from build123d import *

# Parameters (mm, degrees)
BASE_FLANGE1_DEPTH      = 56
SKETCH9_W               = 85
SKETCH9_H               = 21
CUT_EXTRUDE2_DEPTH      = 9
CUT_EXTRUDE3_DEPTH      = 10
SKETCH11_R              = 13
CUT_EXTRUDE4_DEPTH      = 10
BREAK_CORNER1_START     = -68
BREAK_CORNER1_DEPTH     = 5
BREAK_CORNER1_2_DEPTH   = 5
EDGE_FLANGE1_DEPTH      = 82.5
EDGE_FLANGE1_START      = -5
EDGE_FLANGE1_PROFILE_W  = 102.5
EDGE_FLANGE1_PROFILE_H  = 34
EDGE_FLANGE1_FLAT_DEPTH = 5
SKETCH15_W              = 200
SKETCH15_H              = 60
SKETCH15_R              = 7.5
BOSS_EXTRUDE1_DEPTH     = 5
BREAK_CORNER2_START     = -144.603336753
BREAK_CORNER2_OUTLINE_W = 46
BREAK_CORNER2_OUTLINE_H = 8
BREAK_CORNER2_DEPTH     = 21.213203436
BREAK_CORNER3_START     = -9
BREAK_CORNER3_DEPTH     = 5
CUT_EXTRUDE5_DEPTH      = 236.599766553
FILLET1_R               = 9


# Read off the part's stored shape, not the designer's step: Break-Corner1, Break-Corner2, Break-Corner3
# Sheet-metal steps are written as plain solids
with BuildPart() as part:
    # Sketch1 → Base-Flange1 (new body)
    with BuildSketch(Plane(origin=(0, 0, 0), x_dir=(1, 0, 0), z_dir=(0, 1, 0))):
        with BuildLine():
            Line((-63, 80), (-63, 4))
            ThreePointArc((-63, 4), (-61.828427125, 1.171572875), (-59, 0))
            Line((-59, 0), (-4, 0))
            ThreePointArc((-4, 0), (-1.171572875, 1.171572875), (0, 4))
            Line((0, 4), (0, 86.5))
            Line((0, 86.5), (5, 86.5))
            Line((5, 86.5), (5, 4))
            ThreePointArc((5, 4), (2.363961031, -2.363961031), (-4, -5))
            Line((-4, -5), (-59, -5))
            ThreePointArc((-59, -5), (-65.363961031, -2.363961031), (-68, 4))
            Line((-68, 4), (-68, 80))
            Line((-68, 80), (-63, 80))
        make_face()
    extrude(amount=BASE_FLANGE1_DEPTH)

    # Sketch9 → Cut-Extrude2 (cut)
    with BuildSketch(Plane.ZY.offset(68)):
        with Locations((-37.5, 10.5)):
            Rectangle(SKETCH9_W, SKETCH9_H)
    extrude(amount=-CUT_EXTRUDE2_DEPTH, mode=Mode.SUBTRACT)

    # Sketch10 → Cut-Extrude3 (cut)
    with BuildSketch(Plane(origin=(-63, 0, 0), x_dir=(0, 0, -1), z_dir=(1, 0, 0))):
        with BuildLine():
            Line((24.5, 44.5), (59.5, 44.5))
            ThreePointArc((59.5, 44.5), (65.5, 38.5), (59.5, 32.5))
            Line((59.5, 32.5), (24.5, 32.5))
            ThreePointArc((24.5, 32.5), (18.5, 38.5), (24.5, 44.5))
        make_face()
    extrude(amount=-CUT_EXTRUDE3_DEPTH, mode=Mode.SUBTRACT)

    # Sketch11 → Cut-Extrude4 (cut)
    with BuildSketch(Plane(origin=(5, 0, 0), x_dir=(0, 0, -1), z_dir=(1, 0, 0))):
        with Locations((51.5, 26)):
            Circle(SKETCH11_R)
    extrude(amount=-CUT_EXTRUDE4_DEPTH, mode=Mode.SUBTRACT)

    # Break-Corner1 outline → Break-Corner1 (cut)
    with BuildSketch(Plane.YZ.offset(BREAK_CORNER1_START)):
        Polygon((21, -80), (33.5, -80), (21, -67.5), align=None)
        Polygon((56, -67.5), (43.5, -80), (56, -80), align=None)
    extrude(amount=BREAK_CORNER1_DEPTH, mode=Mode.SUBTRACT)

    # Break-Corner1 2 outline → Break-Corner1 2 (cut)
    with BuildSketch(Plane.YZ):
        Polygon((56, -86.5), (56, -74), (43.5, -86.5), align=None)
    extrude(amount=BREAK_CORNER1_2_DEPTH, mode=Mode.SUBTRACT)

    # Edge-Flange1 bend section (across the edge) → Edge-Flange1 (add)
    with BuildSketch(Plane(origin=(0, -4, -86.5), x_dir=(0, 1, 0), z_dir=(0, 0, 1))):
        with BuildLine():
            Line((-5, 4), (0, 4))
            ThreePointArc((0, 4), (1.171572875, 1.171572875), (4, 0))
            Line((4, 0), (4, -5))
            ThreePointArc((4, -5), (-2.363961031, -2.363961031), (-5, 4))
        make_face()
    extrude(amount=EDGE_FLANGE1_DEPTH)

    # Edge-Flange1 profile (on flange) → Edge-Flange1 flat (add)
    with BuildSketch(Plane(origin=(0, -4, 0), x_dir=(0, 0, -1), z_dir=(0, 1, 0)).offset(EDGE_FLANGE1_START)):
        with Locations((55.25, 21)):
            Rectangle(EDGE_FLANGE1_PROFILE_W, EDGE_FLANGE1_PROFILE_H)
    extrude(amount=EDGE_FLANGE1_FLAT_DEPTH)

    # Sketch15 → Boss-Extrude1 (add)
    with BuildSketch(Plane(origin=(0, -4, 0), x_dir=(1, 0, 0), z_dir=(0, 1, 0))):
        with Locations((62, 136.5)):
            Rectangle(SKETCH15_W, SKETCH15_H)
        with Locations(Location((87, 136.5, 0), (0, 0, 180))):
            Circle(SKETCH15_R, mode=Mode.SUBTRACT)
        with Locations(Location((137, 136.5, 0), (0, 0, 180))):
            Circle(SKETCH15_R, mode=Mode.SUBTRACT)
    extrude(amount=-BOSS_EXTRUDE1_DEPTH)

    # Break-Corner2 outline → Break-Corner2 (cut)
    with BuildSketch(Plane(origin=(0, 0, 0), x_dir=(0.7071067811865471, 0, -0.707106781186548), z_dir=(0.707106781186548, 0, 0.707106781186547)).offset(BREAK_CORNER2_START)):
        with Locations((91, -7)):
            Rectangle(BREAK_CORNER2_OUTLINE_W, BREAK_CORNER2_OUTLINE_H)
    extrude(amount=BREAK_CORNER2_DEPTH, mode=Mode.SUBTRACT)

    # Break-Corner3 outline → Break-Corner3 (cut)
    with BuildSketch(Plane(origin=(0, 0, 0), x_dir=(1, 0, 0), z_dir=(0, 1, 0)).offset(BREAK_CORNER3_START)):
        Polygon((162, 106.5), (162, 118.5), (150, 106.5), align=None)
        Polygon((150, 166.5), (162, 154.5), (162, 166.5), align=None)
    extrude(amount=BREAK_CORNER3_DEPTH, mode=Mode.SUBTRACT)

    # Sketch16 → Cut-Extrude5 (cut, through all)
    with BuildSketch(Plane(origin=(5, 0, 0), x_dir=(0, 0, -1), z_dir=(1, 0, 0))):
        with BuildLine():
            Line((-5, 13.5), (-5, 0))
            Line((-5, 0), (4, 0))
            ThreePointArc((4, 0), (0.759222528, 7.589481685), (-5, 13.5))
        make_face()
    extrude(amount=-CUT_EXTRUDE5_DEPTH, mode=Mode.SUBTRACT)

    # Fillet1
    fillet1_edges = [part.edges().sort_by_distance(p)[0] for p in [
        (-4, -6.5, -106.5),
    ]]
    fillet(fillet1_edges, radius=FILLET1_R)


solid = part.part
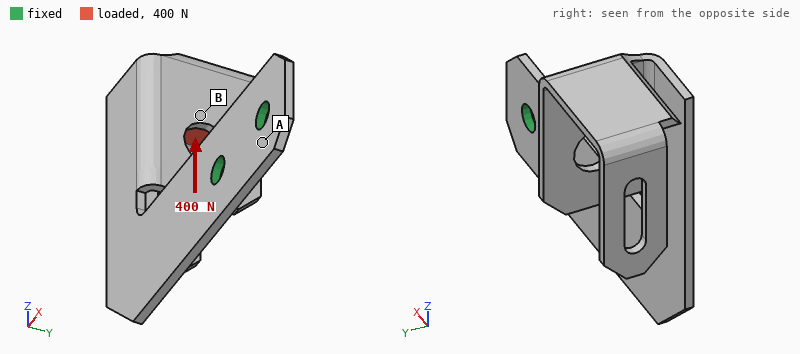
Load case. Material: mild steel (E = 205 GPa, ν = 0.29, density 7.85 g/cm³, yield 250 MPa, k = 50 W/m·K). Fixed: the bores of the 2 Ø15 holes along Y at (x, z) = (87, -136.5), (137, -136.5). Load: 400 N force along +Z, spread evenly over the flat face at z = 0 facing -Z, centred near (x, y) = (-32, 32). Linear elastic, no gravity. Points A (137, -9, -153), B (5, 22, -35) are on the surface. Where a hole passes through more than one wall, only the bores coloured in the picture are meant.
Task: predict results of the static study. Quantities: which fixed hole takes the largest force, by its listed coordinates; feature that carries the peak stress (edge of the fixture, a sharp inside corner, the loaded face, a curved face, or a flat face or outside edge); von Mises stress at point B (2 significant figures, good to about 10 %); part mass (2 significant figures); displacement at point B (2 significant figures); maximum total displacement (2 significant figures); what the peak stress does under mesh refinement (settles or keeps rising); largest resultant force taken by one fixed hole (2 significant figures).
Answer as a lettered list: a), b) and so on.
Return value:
a) (87, -136.5)
b) a sharp inside corner
c) 30 MPa
d) 970 g
e) 1.5 mm
f) 2.5 mm
g) keeps rising
h) 950 N
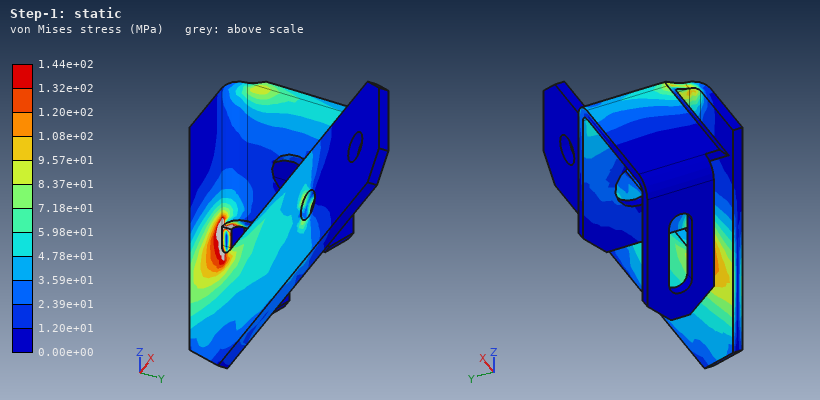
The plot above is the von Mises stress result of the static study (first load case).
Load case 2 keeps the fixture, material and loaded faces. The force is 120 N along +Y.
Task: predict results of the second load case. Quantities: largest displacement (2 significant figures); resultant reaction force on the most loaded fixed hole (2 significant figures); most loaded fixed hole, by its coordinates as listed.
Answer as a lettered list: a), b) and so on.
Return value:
a) 2.9 mm
b) 150 N
c) (87, -136.5)
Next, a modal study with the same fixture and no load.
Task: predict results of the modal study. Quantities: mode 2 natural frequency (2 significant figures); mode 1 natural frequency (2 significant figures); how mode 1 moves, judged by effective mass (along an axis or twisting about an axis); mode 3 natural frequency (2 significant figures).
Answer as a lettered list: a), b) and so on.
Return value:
a) 130 Hz
b) 60 Hz
c) along Y
d) 240 Hz
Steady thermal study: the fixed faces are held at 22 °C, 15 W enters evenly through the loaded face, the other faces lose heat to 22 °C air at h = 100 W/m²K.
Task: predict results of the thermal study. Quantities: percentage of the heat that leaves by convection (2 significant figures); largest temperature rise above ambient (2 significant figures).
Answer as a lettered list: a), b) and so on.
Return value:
a) 100 %
b) 22 K
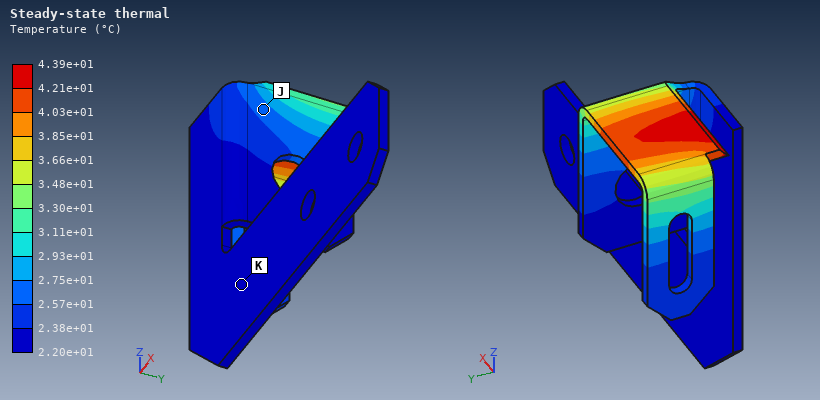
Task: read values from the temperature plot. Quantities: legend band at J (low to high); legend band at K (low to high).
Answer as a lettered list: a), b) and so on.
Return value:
a) 2.57e+01 to 2.75e+01 °C
b) 2.20e+01 to 2.38e+01 °C
